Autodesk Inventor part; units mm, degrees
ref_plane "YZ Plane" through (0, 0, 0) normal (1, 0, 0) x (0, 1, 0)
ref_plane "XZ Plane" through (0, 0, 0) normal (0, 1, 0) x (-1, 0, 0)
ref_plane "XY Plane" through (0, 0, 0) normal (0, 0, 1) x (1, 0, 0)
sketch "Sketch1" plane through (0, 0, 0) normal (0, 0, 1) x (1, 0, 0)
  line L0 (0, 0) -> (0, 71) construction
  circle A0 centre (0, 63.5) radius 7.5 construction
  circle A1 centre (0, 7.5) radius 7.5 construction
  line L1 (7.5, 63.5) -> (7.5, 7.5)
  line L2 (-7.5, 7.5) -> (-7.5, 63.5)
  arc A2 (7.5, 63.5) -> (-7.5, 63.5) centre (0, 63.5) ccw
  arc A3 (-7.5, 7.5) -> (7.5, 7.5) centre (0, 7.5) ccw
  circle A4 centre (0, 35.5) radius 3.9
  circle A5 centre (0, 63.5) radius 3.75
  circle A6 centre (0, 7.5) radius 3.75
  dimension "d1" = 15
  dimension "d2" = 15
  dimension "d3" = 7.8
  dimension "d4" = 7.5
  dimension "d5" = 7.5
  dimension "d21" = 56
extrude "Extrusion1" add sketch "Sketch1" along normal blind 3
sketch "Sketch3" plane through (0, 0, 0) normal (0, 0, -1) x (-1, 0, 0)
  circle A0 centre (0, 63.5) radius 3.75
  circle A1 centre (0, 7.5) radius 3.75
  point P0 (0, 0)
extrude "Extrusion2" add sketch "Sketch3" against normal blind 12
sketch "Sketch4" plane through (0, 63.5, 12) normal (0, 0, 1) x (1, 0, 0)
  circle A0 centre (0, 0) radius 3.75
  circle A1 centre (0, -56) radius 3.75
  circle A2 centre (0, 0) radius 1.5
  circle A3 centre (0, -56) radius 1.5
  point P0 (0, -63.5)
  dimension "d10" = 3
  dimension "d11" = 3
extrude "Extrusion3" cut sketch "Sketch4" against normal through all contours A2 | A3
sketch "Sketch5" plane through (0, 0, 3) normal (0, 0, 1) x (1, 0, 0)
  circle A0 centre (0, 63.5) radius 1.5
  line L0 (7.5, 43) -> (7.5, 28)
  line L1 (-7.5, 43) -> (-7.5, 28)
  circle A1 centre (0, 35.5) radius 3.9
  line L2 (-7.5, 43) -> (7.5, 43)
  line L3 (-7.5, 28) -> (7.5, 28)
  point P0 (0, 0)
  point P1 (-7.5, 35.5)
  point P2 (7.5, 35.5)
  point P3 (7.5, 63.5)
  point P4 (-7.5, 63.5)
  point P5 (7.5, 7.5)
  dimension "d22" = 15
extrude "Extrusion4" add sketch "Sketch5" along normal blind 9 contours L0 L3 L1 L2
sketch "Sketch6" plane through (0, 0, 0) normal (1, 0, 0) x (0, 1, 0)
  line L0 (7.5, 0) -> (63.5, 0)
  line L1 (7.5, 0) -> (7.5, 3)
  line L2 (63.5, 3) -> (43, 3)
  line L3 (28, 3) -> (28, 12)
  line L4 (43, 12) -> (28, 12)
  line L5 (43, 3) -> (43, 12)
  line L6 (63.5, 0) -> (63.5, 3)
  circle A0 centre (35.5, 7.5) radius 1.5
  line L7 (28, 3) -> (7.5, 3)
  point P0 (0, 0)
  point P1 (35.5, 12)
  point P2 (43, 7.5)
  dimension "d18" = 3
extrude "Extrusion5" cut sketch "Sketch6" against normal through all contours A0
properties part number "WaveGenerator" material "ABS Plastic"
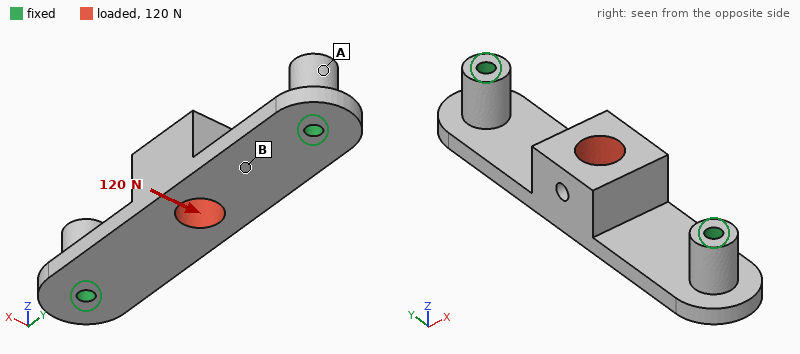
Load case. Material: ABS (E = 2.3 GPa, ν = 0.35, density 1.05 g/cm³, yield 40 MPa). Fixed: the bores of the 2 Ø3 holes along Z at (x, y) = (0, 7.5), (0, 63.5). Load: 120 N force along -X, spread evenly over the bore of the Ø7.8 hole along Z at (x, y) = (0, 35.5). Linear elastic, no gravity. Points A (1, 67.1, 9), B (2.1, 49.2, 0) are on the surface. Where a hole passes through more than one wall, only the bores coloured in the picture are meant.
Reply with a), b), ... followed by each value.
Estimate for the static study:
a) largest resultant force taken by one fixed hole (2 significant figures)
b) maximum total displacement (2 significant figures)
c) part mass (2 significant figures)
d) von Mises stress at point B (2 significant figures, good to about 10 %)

a) 60 N
b) 0.70 mm
c) 5.4 g
d) 7.0 MPa
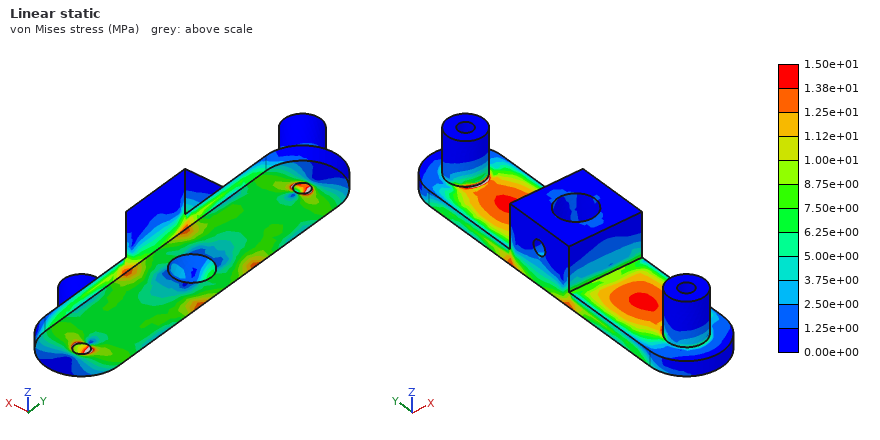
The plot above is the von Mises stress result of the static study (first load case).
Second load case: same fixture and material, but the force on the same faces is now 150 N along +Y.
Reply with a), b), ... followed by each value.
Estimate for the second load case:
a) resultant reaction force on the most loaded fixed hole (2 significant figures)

a) 77 N
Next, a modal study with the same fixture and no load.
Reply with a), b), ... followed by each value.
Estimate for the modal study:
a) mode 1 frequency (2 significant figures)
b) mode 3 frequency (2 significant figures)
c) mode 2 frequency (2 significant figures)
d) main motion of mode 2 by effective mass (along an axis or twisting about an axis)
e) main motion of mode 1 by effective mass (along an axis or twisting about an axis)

a) 1300 Hz
b) 2900 Hz
c) 1500 Hz
d) along X
e) along Z
